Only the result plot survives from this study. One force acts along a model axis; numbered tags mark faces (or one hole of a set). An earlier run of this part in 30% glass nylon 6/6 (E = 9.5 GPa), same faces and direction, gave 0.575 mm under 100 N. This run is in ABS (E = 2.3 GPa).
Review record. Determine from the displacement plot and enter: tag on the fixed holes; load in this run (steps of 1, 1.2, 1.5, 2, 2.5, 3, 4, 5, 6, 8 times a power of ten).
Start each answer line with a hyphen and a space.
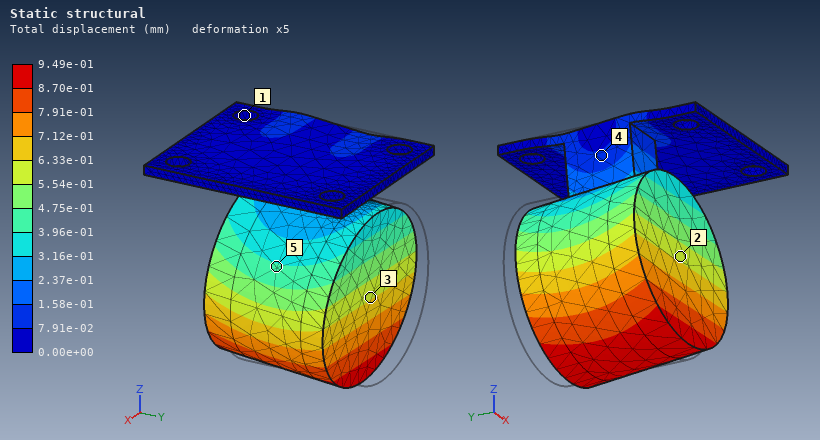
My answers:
- 1
- 40 N
